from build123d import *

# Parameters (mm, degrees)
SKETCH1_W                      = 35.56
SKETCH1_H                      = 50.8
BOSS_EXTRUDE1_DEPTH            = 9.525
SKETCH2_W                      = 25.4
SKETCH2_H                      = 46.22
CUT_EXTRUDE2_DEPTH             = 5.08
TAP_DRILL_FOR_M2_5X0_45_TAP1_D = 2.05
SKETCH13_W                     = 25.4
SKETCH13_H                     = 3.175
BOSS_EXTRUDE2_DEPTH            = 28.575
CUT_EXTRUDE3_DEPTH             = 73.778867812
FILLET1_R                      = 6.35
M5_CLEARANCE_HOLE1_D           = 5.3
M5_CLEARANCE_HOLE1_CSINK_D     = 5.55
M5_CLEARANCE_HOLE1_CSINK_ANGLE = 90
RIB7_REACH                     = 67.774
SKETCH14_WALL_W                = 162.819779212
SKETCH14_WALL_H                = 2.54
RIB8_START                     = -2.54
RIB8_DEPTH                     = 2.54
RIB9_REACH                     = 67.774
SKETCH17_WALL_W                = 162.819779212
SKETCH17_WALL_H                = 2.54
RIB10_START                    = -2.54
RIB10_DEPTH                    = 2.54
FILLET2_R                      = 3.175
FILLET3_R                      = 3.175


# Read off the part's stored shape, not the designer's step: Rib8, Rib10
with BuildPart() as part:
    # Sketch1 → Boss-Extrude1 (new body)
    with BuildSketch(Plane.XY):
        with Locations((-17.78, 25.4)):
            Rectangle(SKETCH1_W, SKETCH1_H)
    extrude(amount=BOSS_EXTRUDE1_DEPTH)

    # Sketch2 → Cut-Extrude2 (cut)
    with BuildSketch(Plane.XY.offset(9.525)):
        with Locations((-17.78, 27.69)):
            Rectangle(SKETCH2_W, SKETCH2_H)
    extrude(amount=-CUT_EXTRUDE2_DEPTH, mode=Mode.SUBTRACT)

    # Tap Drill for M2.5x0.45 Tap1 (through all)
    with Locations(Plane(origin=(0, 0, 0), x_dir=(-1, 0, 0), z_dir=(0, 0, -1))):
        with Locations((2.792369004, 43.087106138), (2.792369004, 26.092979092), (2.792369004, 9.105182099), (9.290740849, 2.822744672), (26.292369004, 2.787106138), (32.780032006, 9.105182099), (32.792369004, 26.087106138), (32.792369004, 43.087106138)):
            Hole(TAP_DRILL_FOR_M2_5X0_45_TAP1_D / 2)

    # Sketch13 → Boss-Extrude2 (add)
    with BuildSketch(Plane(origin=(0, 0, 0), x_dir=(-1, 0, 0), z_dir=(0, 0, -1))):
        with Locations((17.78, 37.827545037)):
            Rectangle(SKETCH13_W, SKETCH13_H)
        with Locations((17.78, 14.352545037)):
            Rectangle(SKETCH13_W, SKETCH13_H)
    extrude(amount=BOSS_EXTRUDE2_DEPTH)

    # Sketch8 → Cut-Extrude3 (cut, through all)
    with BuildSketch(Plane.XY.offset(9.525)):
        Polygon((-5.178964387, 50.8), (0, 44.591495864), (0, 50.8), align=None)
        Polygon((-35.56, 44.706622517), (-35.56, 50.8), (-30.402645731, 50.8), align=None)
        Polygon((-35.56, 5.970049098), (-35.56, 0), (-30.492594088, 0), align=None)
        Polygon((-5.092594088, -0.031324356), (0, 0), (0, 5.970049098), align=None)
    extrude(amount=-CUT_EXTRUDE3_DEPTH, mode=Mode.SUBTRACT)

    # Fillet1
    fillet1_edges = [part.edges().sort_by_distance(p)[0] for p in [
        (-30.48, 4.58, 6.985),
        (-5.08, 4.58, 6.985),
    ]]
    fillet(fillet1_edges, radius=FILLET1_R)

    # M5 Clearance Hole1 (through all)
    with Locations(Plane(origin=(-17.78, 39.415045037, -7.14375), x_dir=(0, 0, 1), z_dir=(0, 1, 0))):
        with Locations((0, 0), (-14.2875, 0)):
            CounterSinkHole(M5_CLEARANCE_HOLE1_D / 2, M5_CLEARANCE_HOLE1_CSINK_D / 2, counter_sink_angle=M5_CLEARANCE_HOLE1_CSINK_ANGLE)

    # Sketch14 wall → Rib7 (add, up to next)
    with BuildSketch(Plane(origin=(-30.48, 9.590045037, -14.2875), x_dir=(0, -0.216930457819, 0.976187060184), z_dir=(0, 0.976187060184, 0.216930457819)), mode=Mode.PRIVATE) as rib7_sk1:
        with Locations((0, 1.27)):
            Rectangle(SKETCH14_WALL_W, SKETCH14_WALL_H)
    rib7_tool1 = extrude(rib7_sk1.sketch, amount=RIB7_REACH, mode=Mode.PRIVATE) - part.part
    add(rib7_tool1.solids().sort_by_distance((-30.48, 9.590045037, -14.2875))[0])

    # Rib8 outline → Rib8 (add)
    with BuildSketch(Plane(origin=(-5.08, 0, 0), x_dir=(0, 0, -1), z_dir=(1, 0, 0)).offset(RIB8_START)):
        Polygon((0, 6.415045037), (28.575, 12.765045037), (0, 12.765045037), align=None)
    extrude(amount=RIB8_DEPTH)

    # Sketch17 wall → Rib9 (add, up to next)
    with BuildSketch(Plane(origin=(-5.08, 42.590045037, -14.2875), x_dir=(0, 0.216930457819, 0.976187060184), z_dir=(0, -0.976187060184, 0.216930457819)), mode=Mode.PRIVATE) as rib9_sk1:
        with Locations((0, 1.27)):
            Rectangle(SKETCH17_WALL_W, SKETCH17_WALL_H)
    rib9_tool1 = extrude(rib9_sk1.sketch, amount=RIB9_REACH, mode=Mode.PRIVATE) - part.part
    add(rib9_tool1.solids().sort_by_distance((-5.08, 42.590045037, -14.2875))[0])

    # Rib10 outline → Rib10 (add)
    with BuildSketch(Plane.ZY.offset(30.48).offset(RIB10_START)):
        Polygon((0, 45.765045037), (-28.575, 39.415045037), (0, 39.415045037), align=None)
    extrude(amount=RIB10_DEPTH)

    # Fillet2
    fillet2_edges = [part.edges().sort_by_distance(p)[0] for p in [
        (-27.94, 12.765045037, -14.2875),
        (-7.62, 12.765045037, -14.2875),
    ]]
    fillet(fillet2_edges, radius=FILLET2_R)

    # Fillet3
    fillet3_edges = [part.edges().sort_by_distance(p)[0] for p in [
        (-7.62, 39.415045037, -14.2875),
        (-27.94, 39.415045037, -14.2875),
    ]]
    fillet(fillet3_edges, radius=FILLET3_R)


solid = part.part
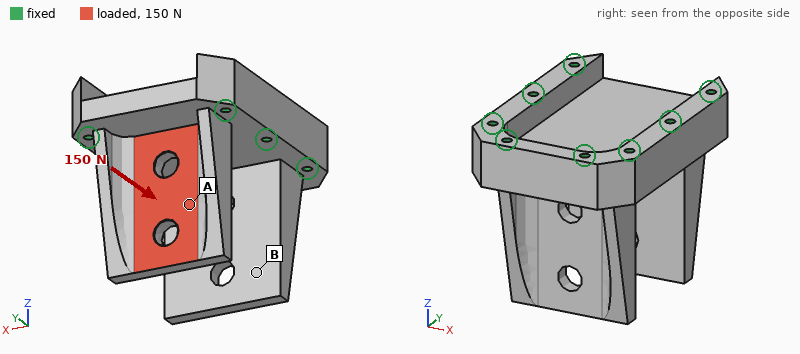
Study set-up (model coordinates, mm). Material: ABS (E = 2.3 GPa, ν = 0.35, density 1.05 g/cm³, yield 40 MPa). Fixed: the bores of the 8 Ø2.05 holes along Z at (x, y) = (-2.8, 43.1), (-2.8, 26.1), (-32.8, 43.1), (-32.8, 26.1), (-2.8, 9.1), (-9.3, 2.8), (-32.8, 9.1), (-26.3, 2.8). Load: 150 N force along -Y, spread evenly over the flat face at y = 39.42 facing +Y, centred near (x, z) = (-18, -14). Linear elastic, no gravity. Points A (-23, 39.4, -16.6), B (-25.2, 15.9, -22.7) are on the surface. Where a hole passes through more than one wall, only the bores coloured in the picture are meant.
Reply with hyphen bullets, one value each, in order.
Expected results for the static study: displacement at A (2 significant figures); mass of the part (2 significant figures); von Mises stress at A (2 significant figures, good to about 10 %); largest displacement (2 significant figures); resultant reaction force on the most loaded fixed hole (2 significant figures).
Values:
- 0.39 mm
- 17 g
- 5.0 MPa
- 0.86 mm
- 75 N
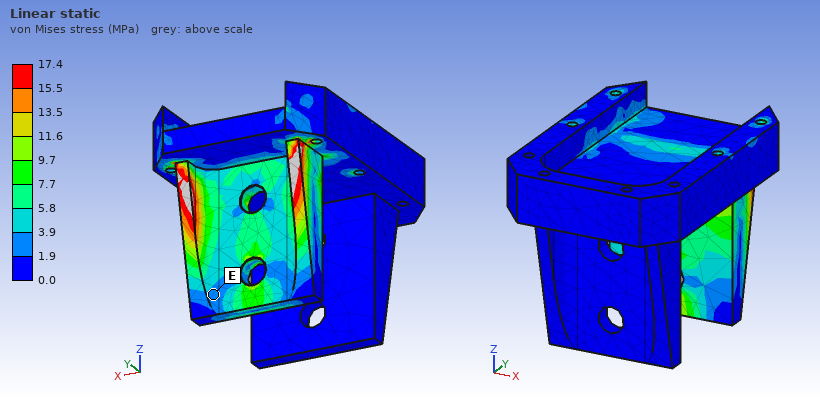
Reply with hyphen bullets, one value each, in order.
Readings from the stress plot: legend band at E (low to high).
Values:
- 1.9 to 3.9 MPa
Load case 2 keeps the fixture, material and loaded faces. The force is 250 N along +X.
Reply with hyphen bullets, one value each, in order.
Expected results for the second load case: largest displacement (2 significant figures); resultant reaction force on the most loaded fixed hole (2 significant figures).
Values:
- 0.31 mm
- 140 N
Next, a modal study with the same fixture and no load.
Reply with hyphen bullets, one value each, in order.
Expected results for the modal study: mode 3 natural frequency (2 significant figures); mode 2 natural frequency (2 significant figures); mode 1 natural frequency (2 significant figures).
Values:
- 2900 Hz
- 1800 Hz
- 1700 Hz
